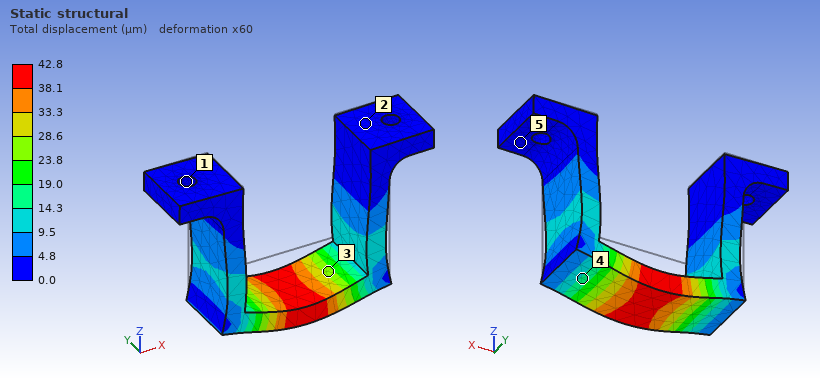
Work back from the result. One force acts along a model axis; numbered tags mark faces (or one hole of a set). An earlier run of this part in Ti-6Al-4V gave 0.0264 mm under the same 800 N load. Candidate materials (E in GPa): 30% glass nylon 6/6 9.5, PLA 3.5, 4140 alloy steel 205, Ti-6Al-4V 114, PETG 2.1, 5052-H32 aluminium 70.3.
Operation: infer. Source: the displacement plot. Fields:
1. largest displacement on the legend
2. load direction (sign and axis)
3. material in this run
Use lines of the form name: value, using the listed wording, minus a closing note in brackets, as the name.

largest displacement on the legend: 42.8 µm
load direction: -Z
material in this run: 5052-H32 aluminium
